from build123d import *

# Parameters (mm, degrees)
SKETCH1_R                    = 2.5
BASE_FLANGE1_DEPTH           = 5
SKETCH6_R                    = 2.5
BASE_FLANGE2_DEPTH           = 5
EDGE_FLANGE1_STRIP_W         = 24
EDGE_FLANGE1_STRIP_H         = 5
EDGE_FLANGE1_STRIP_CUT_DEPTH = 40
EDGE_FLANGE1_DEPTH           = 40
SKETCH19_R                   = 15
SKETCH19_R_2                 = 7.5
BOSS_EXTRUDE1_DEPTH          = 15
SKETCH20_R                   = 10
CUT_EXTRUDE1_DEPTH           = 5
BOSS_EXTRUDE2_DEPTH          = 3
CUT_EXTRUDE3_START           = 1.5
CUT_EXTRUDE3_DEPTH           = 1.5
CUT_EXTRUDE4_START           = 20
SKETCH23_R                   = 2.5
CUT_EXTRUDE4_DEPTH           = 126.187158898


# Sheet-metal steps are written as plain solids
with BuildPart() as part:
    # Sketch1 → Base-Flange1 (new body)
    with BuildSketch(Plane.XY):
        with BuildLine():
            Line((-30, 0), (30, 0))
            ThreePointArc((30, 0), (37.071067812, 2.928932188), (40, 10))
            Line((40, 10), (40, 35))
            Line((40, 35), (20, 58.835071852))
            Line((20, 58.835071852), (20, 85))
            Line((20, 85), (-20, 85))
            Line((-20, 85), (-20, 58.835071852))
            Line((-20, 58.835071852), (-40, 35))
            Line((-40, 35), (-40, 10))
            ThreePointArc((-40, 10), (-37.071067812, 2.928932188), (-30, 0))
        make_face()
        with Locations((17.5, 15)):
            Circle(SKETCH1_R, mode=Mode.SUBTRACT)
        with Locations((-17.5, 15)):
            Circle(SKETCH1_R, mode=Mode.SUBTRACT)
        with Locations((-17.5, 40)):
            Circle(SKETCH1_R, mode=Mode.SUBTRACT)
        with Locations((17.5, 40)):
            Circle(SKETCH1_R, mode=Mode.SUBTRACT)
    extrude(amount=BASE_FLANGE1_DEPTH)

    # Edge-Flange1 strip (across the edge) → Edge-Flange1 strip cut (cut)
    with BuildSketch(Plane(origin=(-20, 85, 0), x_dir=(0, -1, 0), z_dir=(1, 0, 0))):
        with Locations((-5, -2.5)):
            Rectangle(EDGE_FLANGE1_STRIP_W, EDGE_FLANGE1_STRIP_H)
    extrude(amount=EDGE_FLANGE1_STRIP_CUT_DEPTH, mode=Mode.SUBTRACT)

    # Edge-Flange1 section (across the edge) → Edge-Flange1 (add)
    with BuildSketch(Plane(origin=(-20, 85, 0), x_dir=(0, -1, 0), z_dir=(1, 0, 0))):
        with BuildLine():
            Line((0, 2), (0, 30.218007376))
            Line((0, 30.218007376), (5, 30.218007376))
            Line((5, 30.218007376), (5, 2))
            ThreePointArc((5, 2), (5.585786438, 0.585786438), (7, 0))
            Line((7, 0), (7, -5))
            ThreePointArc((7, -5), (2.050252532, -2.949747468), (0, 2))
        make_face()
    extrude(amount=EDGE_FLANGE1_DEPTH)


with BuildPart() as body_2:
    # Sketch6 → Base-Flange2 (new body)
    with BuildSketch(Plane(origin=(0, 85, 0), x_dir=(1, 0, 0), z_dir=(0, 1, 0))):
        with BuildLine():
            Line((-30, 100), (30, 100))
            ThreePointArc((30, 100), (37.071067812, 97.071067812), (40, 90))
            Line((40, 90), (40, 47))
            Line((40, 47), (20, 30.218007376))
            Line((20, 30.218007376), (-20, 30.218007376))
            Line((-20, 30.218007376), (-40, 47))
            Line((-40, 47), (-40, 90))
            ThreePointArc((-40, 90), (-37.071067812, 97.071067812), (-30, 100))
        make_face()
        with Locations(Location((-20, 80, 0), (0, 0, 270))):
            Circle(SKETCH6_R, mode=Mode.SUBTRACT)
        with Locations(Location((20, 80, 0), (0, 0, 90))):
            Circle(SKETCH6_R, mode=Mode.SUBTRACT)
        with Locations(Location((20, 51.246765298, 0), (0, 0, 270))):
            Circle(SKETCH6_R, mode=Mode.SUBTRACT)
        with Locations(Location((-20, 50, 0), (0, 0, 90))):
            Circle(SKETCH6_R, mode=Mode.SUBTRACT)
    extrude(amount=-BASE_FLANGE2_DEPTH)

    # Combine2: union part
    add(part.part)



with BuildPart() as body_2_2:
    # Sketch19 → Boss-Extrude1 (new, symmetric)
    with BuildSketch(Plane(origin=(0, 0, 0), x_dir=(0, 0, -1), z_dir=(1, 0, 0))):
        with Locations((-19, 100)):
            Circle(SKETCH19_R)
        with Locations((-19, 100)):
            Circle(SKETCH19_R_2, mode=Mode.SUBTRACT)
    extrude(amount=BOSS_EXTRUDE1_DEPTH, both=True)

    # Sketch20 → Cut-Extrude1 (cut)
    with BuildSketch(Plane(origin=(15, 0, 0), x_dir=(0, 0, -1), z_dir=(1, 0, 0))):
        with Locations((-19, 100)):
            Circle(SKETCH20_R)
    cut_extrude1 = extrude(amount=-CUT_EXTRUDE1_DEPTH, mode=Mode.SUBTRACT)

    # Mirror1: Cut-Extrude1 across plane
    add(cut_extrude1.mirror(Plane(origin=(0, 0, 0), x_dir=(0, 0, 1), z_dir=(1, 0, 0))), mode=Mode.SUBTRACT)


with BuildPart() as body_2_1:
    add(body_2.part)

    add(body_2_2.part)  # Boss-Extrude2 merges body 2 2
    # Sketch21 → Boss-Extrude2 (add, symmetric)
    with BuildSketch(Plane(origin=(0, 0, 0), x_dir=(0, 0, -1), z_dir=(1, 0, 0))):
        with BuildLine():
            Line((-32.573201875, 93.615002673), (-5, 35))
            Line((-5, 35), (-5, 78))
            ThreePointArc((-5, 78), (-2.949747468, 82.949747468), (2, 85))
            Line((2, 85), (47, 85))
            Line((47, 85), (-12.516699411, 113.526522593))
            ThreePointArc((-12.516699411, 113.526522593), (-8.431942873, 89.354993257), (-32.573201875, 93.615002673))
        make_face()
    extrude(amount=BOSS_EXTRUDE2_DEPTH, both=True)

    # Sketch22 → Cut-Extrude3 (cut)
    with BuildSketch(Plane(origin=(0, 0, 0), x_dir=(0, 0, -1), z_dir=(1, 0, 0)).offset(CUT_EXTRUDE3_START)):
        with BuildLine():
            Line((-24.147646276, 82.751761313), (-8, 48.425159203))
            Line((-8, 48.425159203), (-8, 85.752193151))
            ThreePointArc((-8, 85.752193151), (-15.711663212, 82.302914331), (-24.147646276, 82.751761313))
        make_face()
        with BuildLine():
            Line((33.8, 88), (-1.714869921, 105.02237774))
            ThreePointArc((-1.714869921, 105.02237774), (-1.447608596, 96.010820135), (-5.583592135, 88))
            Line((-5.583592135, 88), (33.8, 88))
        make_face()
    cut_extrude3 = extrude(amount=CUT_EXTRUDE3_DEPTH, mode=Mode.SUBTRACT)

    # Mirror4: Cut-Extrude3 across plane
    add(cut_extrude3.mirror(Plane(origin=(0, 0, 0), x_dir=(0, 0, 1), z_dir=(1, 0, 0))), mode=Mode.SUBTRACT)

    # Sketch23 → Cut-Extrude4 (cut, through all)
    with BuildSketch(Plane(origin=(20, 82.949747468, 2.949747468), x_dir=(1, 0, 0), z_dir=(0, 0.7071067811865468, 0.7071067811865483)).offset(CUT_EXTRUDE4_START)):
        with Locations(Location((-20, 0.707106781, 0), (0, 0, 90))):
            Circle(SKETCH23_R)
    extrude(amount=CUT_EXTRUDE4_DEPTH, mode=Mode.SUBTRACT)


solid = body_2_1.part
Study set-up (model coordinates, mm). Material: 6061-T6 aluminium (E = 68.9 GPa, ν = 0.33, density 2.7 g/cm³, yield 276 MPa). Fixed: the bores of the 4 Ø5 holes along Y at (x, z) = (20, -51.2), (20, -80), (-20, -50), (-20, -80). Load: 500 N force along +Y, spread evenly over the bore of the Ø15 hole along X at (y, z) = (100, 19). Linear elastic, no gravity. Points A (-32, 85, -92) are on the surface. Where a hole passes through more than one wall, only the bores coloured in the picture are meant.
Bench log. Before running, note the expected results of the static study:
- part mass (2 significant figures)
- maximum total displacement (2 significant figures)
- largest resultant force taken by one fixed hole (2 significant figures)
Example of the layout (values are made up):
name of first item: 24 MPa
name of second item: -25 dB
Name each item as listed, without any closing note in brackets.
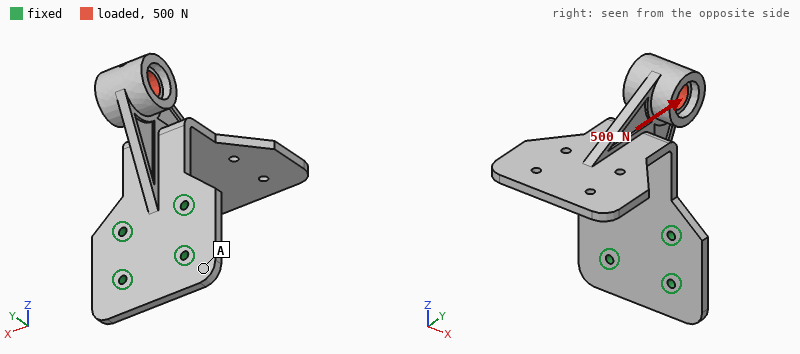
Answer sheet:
part mass: 210 g
maximum total displacement: 1.4 mm
largest resultant force taken by one fixed hole: 500 N
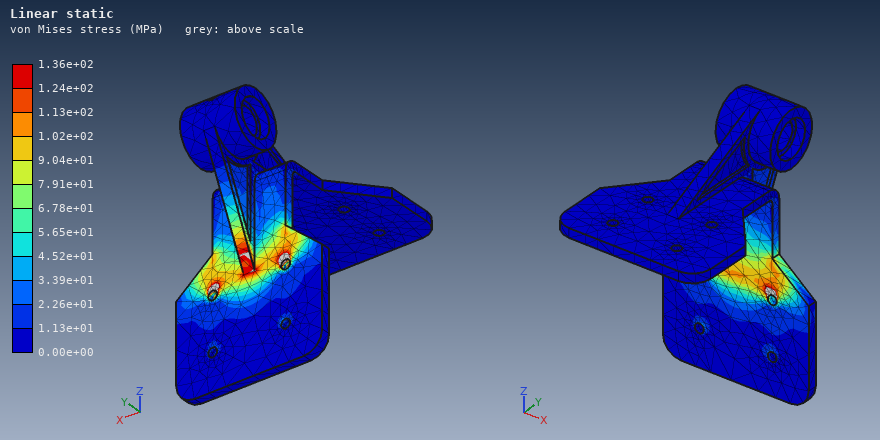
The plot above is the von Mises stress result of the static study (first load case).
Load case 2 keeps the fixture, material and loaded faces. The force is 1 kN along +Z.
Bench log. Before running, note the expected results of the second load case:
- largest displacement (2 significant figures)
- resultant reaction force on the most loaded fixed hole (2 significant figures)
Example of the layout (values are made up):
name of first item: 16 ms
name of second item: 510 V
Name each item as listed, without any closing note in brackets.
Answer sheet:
largest displacement: 0.81 mm
resultant reaction force on the most loaded fixed hole: 360 N
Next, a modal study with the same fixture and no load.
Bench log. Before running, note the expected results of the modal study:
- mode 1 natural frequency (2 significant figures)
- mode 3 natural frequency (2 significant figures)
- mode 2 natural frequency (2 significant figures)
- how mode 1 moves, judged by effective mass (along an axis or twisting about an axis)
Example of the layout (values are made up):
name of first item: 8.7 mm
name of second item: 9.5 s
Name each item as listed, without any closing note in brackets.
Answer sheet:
mode 1 natural frequency: 310 Hz
mode 3 natural frequency: 1100 Hz
mode 2 natural frequency: 400 Hz
how mode 1 moves, judged by effective mass: along Y
